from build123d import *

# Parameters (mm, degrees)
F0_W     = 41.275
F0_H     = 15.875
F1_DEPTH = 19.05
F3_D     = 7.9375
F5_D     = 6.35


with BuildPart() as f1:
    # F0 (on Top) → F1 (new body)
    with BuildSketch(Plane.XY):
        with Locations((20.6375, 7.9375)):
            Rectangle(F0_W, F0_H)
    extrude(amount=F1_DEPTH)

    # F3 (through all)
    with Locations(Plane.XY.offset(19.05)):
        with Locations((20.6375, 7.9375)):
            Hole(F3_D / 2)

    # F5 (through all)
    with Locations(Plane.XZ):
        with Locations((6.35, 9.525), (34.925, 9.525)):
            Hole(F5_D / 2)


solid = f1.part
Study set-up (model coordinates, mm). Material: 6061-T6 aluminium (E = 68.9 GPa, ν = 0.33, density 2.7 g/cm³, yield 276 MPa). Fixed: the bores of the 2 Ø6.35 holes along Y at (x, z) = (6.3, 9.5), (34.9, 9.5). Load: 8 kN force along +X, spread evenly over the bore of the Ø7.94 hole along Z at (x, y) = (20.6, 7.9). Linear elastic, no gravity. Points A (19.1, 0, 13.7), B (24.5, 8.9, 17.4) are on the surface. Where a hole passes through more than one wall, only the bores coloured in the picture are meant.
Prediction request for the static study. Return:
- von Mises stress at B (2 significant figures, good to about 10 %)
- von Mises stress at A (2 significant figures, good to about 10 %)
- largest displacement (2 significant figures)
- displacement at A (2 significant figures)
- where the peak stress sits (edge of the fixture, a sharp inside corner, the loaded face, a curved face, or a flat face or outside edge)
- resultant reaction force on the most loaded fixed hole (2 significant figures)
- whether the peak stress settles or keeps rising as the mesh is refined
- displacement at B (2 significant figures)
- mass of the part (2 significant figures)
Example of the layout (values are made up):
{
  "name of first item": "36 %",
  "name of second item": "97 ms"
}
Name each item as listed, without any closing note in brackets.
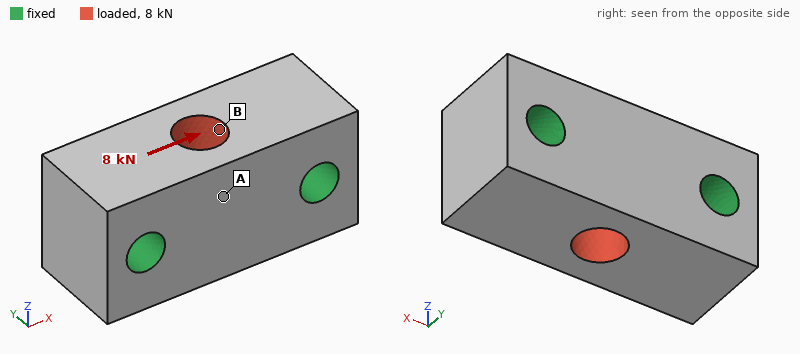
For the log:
{
  "von Mises stress at B": "18 MPa",
  "von Mises stress at A": "4.9 MPa",
  "largest displacement": "3.2 µm",
  "displacement at A": "1.9 µm",
  "where the peak stress sits": "edge of the fixture",
  "resultant reaction force on the most loaded fixed hole": "4.0 kN",
  "whether the peak stress settles or keeps rising as the mesh is refined": "keeps rising",
  "displacement at B": "3.0 µm",
  "mass of the part": "28 g"
}
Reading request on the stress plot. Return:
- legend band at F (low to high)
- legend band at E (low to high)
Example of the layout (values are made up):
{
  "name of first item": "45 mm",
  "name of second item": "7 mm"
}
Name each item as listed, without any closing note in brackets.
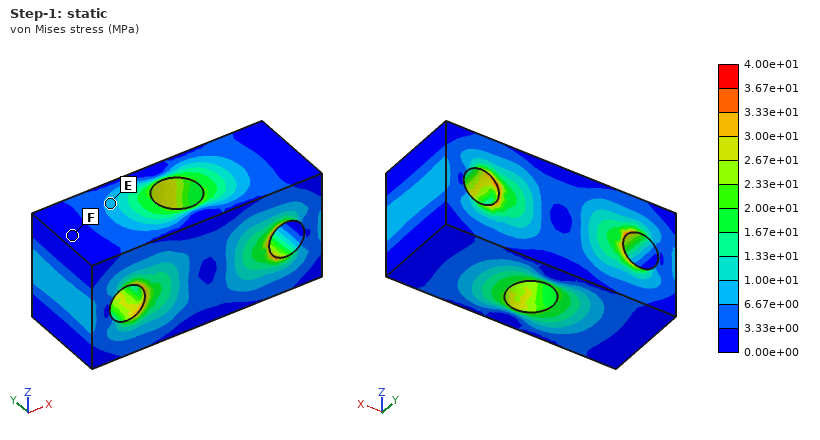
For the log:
{
  "legend band at F": "0.00e+00 to 3.33e+00 MPa",
  "legend band at E": "6.67e+00 to 1.00e+01 MPa"
}
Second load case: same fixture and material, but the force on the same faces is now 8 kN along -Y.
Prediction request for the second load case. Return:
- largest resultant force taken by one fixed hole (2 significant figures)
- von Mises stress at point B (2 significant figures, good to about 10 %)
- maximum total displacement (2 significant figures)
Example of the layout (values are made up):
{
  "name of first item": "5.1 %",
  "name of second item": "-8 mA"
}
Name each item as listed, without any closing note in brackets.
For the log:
{
  "largest resultant force taken by one fixed hole": "4.0 kN",
  "von Mises stress at point B": "34 MPa",
  "maximum total displacement": "10 µm"
}
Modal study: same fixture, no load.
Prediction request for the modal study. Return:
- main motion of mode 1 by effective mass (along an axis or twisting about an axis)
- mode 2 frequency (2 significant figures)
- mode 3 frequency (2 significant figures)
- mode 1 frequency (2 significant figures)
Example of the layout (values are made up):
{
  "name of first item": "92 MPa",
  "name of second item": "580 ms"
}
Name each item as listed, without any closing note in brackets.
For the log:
{
  "main motion of mode 1 by effective mass": "along Z",
  "mode 2 frequency": "53 kHz",
  "mode 3 frequency": "53 kHz",
  "mode 1 frequency": "47 kHz"
}
